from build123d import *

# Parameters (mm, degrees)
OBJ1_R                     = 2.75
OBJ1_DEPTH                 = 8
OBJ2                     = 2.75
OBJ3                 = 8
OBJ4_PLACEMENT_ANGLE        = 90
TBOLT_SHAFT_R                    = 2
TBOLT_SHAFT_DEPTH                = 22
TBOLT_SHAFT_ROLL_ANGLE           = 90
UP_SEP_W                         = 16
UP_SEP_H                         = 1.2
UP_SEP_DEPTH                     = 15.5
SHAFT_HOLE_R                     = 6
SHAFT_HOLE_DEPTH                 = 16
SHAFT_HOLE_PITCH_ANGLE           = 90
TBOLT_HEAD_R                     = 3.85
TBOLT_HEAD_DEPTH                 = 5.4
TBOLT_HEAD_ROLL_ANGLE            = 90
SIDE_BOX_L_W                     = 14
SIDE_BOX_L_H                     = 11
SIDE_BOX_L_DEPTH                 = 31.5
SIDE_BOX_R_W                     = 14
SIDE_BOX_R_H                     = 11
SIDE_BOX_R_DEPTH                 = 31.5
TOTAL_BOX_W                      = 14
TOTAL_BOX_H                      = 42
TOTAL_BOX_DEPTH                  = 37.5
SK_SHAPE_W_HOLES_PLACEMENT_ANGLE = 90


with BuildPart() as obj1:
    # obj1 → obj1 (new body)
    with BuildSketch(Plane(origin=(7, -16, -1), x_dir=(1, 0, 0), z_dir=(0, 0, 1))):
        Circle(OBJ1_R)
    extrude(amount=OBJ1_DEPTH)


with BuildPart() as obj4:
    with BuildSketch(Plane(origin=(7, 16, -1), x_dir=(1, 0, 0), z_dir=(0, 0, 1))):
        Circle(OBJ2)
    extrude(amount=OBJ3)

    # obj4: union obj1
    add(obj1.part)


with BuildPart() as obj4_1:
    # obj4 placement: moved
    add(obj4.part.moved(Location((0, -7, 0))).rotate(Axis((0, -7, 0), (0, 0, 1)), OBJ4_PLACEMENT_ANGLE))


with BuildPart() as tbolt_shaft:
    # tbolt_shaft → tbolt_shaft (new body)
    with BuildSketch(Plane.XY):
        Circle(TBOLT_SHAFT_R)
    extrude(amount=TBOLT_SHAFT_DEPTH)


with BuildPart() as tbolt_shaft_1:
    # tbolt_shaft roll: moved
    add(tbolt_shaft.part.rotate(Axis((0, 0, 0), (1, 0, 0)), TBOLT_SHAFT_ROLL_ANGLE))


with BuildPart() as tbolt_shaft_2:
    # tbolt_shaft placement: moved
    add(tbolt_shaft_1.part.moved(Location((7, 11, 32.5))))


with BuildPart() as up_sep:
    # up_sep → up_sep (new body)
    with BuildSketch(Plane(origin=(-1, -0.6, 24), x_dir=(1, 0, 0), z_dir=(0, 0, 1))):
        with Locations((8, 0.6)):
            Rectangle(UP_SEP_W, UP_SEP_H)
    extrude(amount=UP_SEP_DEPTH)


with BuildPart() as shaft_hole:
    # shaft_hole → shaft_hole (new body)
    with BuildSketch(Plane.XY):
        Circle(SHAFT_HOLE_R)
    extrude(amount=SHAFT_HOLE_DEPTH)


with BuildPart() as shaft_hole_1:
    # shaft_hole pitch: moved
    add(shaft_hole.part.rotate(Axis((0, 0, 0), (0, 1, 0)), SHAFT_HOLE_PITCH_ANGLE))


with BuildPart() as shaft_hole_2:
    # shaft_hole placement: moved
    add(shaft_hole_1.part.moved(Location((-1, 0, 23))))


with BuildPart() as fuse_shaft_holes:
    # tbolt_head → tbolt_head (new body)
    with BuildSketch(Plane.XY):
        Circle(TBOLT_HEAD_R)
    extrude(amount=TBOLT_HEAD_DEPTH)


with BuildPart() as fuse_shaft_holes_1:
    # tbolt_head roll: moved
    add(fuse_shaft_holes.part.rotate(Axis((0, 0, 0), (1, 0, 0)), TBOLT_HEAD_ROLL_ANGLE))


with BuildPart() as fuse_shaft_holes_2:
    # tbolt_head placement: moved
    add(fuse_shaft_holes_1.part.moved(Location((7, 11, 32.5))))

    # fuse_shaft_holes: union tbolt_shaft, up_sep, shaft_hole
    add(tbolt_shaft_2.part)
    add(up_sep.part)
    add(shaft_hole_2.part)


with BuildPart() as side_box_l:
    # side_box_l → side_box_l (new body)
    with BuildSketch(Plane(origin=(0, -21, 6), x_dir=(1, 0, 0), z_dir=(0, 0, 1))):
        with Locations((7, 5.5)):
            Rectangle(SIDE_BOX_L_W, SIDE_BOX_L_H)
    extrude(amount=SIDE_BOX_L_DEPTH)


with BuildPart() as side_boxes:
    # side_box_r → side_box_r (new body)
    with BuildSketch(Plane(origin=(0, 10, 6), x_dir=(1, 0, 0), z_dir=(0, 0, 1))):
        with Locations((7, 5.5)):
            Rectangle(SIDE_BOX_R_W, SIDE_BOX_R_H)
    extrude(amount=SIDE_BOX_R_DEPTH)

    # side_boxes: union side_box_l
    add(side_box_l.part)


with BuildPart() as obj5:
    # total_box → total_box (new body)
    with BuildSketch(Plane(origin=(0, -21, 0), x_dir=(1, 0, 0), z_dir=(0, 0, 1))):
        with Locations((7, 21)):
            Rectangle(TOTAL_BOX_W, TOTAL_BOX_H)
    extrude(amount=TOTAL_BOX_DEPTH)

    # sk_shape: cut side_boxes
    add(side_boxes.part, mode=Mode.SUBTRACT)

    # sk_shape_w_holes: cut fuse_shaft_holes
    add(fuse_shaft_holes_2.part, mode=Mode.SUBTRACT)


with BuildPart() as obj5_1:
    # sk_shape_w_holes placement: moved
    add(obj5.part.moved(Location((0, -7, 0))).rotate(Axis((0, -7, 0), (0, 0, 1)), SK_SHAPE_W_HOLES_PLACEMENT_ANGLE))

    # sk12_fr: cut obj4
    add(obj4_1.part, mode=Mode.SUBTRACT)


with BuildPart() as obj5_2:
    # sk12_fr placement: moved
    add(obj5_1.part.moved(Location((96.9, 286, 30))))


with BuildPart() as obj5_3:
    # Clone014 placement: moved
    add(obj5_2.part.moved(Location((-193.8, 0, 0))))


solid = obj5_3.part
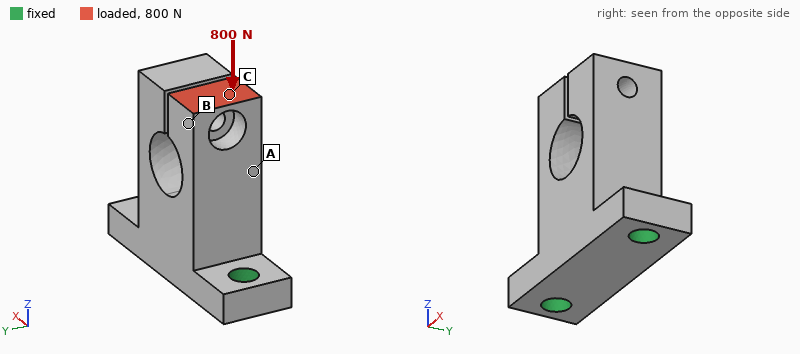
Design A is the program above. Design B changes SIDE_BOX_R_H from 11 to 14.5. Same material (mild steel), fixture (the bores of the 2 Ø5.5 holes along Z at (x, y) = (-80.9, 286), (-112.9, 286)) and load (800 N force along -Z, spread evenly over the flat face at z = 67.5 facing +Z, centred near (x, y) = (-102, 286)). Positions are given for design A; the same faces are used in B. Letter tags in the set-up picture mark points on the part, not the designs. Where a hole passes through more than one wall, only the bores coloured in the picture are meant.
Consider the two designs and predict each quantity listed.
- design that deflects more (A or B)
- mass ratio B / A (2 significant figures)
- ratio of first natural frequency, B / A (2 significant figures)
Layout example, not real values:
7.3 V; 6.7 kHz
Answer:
B; 0.93; 0.80
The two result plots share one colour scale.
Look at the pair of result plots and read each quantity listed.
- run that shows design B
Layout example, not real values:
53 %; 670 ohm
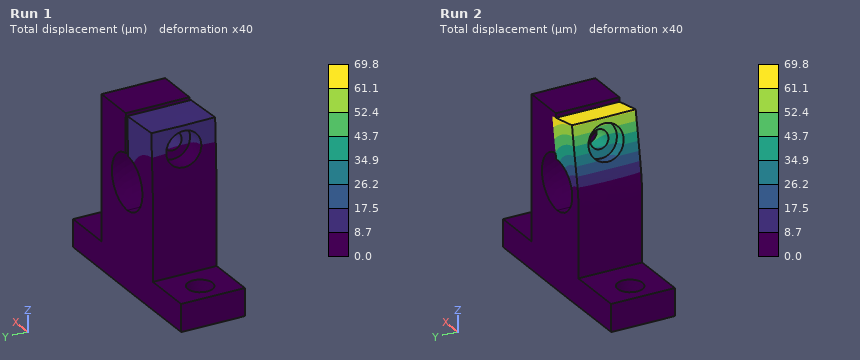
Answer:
Run 2
